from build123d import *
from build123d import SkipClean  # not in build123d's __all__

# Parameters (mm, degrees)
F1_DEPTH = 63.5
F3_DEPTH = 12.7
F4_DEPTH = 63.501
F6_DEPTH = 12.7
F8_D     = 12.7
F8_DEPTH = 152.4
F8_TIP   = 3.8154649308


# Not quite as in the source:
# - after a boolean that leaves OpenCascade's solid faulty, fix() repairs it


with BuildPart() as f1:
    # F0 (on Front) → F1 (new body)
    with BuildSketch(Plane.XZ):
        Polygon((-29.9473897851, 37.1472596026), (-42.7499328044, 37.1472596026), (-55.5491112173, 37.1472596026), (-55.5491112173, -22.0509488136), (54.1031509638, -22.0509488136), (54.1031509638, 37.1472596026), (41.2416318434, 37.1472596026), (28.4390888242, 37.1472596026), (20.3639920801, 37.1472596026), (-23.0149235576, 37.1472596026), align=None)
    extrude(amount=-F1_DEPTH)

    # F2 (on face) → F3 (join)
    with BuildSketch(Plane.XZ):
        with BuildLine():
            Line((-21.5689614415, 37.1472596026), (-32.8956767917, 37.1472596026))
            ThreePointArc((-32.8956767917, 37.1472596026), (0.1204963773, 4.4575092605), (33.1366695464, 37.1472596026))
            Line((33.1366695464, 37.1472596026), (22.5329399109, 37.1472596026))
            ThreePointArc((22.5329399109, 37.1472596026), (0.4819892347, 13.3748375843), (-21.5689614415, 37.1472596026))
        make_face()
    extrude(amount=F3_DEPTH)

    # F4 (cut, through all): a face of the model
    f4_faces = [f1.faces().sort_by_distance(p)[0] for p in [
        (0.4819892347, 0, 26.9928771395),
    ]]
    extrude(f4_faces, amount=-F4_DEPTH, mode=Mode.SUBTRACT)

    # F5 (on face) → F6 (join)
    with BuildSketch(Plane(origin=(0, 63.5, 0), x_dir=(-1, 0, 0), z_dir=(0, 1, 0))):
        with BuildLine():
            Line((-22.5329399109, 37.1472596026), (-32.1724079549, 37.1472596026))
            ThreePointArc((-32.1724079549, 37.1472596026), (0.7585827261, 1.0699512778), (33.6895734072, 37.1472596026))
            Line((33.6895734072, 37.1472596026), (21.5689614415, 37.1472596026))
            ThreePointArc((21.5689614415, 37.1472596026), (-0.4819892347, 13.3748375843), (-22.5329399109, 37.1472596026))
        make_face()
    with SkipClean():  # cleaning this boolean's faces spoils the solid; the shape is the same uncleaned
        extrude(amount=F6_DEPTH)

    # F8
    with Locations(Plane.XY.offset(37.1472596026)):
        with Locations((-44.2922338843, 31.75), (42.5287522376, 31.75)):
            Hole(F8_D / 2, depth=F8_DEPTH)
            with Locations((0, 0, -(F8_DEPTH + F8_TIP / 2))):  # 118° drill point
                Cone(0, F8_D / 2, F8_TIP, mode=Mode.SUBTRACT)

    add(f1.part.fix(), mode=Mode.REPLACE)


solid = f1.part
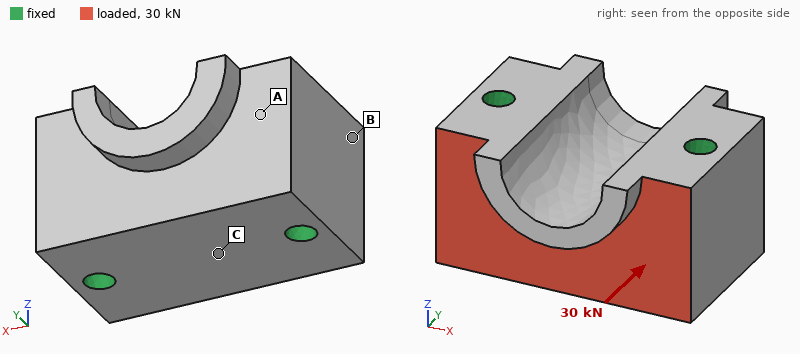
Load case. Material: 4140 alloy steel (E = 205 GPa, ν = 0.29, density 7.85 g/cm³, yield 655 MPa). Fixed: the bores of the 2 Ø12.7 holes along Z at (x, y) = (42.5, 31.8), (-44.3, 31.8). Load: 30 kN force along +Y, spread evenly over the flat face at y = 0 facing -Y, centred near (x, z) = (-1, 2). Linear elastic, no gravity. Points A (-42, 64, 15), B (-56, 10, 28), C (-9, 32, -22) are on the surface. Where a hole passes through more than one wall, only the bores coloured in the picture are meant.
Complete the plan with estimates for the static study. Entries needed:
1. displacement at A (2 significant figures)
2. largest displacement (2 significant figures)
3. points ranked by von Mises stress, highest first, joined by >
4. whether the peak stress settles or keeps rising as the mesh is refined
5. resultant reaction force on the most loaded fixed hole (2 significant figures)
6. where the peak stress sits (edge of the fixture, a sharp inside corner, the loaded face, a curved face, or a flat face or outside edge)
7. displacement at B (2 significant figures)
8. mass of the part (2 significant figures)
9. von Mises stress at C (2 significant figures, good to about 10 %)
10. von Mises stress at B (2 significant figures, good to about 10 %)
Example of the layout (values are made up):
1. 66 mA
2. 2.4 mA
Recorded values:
1. 0.57 µm
2. 2.6 µm
3. B > C > A
4. keeps rising
5. 15 kN
6. edge of the fixture
7. 0.47 µm
8. 2.9 kg
9. 3.4 MPa
10. 6.2 MPa
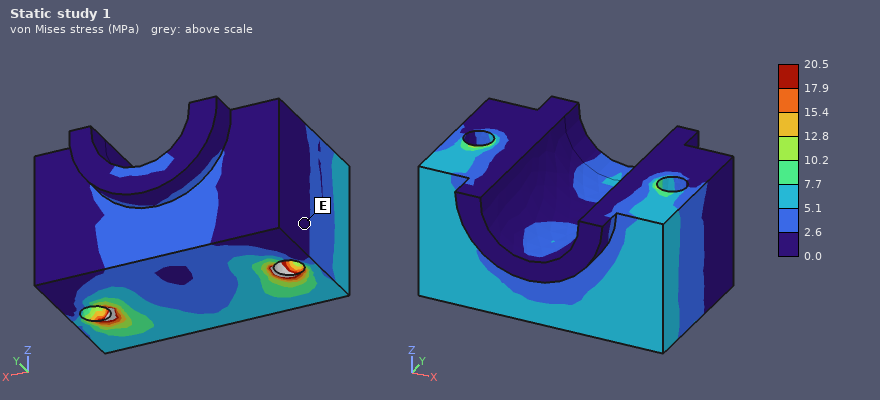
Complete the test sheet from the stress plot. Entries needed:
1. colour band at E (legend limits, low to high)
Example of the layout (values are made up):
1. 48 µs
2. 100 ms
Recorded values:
1. 0.0 to 2.6 MPa
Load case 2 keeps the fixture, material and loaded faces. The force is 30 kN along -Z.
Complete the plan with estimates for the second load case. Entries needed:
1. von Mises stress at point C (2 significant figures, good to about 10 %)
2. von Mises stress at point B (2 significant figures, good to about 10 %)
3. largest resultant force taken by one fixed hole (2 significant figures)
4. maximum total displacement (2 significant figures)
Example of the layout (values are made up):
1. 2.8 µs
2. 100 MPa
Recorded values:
1. 7.3 MPa
2. 11 MPa
3. 15 kN
4. 6.8 µm
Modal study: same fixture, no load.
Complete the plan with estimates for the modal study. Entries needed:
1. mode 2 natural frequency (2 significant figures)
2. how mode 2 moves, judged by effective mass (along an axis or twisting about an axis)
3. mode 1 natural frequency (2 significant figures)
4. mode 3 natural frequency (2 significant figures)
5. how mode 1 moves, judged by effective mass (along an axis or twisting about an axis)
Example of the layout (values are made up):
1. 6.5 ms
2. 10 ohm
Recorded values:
1. 13 kHz
2. along Z
3. 13 kHz
4. 15 kHz
5. along Y
